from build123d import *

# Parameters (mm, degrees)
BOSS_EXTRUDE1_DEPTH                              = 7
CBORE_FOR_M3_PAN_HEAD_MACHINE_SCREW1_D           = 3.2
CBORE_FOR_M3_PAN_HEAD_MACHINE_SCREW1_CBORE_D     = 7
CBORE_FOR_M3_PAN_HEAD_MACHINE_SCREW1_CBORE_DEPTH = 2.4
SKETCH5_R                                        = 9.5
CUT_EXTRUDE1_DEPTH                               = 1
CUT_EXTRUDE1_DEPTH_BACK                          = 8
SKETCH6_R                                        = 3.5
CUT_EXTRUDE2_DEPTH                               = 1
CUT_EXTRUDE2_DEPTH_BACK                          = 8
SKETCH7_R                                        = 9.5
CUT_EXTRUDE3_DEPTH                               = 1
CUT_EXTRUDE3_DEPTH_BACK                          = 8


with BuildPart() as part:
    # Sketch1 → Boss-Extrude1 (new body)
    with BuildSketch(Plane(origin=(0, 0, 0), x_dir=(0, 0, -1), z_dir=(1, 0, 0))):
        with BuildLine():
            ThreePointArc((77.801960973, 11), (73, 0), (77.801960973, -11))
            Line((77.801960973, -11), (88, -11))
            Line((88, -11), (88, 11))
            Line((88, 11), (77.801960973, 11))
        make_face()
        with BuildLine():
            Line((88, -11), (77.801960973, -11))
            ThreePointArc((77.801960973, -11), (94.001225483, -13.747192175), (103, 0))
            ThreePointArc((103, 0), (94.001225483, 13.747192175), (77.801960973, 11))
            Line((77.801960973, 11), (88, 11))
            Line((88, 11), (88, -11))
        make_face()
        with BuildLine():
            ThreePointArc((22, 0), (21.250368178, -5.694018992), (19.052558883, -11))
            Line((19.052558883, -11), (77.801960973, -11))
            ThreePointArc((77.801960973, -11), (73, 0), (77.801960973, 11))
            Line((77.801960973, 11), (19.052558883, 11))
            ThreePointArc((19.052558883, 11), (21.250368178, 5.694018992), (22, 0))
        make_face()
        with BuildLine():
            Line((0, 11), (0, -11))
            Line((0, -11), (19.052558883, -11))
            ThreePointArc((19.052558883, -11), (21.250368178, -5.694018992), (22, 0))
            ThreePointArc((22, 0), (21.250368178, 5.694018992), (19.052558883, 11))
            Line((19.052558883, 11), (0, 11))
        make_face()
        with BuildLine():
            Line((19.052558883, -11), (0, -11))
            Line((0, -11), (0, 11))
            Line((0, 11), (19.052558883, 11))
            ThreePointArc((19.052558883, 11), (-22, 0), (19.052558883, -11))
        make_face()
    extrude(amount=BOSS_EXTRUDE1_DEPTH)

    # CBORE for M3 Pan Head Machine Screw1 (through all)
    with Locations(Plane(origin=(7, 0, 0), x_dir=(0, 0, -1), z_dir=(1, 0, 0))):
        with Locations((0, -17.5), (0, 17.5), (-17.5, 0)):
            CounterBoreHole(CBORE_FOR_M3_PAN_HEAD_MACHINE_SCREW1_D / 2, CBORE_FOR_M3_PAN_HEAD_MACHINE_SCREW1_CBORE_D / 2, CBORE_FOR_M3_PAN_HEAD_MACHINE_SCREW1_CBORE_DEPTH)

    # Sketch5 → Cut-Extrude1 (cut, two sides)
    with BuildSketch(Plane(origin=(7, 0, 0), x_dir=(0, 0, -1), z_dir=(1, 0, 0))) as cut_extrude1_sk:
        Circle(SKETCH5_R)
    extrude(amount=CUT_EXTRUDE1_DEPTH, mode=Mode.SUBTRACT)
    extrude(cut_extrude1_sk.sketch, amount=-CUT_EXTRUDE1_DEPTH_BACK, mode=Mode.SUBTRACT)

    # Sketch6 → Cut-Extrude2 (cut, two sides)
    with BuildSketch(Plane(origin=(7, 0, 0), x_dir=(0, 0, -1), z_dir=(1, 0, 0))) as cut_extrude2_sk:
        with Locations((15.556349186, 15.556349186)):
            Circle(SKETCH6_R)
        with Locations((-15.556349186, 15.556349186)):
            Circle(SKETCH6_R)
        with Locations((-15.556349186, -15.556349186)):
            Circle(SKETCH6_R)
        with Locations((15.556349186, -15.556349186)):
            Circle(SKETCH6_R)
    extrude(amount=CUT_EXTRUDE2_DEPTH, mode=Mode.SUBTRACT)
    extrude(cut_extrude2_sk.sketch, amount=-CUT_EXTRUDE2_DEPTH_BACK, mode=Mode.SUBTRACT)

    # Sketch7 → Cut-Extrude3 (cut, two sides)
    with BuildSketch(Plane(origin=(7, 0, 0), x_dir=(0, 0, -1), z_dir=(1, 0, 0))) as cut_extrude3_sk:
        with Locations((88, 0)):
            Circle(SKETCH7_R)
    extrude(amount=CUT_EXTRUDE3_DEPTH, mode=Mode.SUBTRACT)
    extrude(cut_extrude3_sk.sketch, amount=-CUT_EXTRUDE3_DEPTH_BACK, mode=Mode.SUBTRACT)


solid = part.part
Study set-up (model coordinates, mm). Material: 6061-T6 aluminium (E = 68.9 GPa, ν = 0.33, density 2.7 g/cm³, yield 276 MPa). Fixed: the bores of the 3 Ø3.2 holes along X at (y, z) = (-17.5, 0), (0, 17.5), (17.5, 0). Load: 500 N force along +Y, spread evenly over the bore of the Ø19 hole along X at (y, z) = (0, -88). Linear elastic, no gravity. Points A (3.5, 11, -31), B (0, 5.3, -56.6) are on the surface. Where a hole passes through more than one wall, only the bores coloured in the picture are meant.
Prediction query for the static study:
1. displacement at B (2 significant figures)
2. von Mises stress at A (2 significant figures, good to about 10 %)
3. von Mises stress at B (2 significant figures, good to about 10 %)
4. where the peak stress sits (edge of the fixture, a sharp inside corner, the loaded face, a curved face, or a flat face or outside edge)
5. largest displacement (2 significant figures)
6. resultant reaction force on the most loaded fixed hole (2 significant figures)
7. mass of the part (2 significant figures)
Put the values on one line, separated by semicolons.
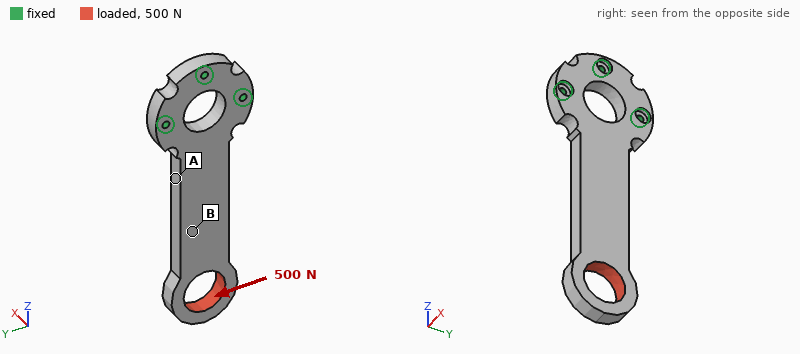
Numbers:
0.11 mm; 50 MPa; 15 MPa; a curved face; 0.32 mm; 1.3 kN; 51 g
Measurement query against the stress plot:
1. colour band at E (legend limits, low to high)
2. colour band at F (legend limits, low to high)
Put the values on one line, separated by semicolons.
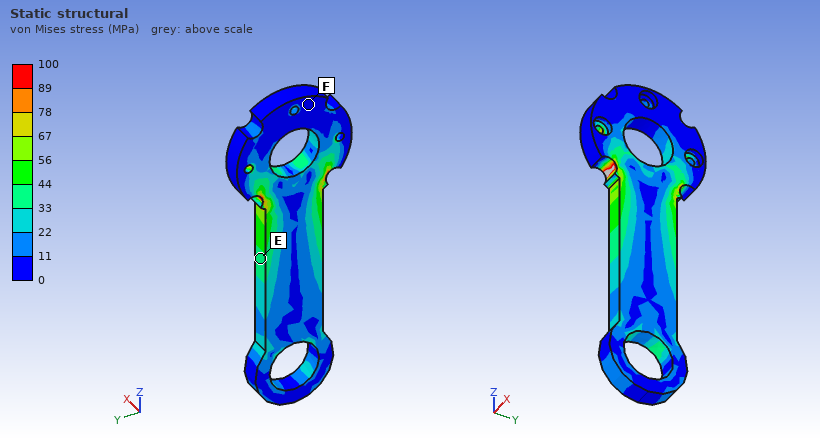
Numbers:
33 to 44 MPa; 0 to 11 MPa
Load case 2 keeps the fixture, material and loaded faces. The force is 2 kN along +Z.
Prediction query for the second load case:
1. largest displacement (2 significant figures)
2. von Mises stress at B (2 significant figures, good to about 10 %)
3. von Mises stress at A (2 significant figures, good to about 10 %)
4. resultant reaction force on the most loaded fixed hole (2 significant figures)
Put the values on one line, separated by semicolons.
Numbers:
50 µm; 13 MPa; 13 MPa; 1.0 kN
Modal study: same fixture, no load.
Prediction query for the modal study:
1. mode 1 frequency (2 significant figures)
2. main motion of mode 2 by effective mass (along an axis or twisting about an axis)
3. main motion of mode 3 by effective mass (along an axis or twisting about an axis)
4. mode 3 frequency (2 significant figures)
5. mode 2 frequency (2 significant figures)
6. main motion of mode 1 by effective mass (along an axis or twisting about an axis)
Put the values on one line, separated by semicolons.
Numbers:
550 Hz; along Y; along X; 3100 Hz; 2100 Hz; along X
